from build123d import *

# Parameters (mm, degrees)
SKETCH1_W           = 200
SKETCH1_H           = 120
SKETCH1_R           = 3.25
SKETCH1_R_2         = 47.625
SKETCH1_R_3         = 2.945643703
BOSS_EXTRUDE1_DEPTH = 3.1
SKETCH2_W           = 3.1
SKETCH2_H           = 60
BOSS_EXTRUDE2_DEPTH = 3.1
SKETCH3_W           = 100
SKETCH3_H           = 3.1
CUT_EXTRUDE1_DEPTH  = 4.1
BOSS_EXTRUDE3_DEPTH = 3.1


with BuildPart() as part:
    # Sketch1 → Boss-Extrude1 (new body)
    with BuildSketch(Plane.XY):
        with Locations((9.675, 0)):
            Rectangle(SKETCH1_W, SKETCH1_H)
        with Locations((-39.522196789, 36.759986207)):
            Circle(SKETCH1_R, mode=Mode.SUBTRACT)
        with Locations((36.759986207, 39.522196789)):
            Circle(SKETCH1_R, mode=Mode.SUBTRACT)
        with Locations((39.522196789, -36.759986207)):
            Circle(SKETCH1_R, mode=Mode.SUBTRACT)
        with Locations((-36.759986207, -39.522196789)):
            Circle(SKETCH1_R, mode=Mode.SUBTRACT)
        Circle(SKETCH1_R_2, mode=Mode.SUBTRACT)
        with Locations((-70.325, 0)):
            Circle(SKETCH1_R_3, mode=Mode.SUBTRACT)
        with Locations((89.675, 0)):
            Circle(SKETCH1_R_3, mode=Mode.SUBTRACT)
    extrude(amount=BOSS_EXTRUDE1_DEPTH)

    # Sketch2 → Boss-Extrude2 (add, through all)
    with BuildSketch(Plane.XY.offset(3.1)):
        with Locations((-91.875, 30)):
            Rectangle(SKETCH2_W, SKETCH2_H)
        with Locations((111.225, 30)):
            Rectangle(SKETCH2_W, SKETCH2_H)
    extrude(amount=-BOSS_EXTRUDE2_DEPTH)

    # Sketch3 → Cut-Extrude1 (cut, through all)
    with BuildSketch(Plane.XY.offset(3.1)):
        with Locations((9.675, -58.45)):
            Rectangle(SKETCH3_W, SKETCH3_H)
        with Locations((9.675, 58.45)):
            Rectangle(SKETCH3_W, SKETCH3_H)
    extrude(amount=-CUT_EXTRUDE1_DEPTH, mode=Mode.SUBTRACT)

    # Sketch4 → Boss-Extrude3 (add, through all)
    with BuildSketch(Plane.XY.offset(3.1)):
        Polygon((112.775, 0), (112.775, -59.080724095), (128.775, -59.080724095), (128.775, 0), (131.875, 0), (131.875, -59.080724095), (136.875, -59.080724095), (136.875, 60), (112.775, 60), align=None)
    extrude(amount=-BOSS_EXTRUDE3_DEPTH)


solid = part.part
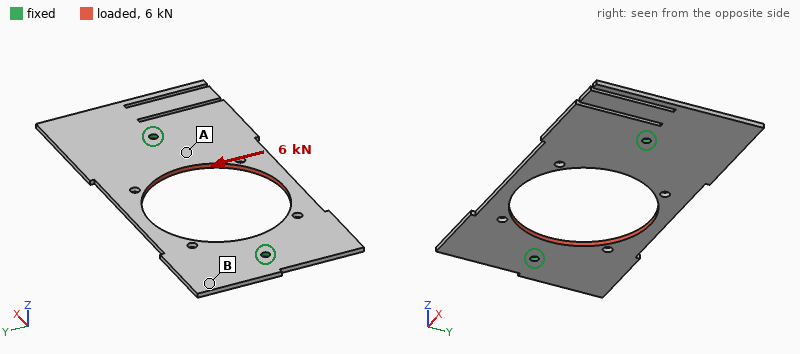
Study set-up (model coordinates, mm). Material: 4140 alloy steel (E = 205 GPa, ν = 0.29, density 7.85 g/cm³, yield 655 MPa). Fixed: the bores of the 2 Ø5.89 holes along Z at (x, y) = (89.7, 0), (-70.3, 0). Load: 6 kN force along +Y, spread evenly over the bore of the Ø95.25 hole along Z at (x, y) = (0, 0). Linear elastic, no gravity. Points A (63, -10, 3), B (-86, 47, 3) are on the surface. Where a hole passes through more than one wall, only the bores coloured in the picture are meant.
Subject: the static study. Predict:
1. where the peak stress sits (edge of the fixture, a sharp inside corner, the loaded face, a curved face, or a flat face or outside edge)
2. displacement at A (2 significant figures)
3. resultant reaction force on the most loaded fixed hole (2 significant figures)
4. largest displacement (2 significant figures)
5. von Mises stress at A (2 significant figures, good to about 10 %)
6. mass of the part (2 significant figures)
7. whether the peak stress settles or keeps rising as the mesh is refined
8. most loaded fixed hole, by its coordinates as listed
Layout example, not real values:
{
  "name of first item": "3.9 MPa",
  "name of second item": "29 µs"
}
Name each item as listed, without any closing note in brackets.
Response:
{
  "where the peak stress sits": "edge of the fixture",
  "displacement at A": "14 µm",
  "resultant reaction force on the most loaded fixed hole": "3.3 kN",
  "largest displacement": "36 µm",
  "von Mises stress at A": "19 MPa",
  "mass of the part": "470 g",
  "whether the peak stress settles or keeps rising as the mesh is refined": "keeps rising",
  "most loaded fixed hole, by its coordinates as listed": "(-70.3, 0)"
}
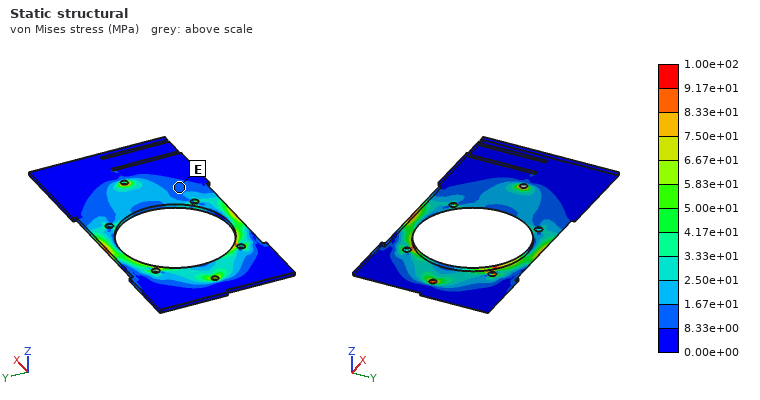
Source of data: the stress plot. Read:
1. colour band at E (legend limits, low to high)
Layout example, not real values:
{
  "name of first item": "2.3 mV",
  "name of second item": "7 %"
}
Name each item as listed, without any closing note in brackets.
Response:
{
  "colour band at E": "8.33e+00 to 1.67e+01 MPa"
}
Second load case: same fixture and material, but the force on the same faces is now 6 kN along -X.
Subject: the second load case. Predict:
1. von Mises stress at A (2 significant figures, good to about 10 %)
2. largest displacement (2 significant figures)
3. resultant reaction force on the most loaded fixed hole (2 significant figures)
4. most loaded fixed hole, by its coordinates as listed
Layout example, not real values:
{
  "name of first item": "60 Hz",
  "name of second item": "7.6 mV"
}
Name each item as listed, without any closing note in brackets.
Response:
{
  "von Mises stress at A": "18 MPa",
  "largest displacement": "14 µm",
  "resultant reaction force on the most loaded fixed hole": "3.3 kN",
  "most loaded fixed hole, by its coordinates as listed": "(89.7, 0)"
}
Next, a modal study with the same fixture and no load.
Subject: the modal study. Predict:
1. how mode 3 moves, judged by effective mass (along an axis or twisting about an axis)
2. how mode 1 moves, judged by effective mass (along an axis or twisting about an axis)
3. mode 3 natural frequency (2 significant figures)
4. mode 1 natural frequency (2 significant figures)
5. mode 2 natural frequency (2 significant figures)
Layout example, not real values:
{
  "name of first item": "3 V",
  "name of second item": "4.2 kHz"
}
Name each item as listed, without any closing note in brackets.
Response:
{
  "how mode 3 moves, judged by effective mass": "along Z",
  "how mode 1 moves, judged by effective mass": "twisting about X",
  "mode 3 natural frequency": "510 Hz",
  "mode 1 natural frequency": "400 Hz",
  "mode 2 natural frequency": "460 Hz"
}
